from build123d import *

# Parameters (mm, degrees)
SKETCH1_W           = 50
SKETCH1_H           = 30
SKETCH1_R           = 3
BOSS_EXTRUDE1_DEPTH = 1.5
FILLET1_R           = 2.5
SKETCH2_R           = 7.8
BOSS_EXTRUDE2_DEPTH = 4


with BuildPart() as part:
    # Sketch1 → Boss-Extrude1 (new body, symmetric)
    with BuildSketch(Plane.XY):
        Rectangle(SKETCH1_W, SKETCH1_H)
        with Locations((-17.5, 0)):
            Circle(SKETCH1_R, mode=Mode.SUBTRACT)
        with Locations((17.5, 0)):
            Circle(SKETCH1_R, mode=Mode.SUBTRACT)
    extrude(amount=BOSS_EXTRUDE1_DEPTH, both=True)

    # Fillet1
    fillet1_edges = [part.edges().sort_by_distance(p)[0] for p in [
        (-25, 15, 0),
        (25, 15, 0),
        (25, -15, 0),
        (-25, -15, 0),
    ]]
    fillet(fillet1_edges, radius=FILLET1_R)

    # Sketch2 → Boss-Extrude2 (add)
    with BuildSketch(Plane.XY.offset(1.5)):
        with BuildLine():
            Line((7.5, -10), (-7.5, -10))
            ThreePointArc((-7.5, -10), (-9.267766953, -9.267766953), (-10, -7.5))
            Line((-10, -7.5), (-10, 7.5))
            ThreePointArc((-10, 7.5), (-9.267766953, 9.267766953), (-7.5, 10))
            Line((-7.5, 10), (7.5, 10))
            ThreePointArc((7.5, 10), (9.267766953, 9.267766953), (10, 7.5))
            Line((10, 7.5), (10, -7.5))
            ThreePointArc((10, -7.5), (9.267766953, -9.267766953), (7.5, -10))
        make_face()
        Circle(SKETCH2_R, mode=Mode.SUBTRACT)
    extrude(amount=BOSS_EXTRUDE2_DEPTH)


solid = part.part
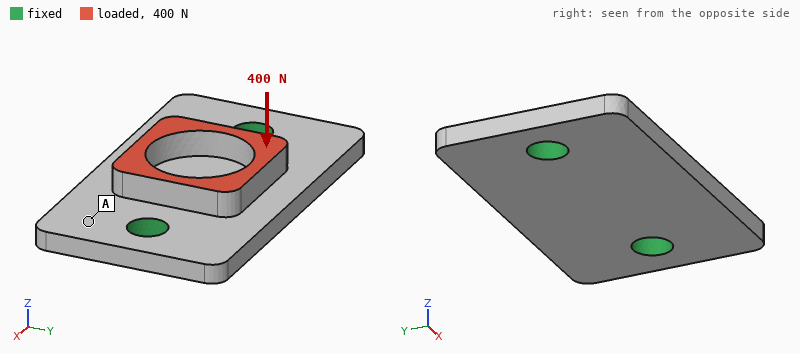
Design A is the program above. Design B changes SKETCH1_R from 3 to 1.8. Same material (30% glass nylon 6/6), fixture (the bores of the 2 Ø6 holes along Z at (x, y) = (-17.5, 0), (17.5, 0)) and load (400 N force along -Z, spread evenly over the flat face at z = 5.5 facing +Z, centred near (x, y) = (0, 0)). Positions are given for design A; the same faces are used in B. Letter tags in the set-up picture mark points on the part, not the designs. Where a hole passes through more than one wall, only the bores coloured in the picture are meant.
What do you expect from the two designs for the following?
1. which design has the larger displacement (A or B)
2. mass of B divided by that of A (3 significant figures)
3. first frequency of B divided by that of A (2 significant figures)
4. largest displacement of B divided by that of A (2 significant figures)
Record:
B
1.02
0.79
1.4
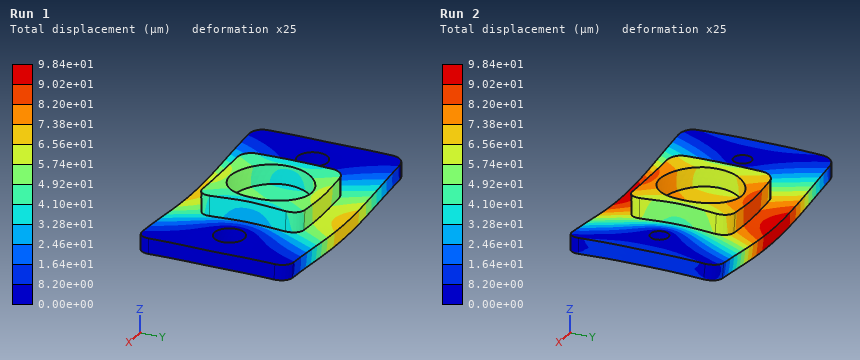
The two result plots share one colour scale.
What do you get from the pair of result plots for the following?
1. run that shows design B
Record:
Run 2
